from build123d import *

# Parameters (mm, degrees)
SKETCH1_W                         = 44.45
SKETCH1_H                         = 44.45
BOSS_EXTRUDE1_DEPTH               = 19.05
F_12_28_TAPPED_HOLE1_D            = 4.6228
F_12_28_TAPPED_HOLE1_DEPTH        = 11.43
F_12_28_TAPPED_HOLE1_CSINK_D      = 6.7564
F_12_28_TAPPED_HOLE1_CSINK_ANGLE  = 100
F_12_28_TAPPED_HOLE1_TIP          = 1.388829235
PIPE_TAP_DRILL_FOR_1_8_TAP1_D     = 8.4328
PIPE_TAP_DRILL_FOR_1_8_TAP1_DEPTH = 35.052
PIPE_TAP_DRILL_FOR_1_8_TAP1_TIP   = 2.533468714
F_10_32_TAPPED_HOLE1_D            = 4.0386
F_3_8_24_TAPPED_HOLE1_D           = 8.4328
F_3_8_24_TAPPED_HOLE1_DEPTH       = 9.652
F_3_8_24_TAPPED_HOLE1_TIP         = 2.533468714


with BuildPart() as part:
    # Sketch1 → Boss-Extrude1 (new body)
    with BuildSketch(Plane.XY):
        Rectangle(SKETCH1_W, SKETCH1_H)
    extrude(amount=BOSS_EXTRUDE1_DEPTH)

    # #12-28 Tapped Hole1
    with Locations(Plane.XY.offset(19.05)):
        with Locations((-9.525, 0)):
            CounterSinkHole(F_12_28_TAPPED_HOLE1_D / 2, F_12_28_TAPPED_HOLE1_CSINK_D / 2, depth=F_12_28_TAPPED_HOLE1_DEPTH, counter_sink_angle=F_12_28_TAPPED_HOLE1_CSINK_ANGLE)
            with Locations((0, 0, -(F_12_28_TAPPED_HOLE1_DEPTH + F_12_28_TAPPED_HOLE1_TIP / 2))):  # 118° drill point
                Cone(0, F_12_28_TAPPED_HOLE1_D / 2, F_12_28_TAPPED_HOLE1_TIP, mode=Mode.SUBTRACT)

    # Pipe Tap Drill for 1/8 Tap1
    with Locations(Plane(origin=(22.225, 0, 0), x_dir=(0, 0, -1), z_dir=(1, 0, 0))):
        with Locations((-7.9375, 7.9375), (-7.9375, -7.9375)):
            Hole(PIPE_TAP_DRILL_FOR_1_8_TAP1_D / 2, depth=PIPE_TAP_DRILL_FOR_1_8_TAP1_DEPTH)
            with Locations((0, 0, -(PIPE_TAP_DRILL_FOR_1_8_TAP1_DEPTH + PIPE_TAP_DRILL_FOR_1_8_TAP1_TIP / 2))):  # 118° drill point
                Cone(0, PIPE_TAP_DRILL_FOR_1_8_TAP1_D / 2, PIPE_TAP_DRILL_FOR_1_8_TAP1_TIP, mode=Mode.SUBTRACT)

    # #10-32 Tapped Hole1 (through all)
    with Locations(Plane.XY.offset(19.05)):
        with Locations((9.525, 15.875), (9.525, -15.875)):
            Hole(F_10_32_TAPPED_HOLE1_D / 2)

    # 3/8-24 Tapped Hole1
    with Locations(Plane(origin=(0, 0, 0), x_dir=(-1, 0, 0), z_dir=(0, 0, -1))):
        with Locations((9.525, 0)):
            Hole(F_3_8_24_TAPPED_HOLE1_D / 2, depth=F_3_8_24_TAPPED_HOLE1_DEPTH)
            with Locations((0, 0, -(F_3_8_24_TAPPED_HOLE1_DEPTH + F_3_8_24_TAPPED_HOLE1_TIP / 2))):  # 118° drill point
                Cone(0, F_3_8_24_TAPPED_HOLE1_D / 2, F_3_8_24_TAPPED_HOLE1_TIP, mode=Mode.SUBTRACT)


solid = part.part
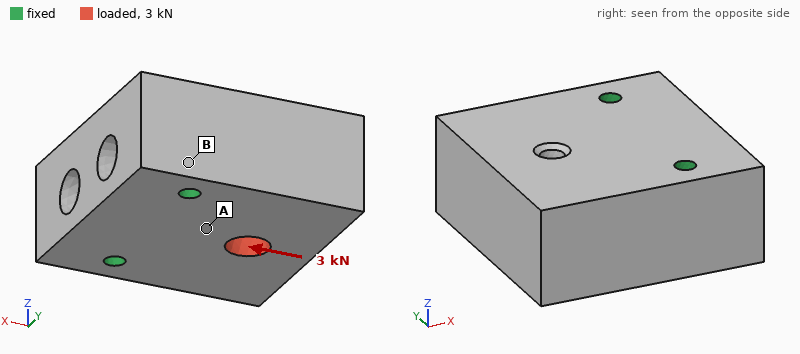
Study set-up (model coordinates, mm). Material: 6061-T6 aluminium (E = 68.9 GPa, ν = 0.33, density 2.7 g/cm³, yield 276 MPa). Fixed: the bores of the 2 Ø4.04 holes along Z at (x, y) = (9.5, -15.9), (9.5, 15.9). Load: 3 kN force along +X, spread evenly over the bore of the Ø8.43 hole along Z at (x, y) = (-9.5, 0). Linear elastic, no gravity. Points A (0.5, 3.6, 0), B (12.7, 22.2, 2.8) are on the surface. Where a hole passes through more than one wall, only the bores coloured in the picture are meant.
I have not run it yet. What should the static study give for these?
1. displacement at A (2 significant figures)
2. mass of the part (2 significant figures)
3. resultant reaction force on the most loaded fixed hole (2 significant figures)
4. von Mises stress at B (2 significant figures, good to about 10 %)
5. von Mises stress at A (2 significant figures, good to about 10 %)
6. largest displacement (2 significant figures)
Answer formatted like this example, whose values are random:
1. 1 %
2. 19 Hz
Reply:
1. 3.8 µm
2. 88 g
3. 1.5 kN
4. 4.7 MPa
5. 11 MPa
6. 8.9 µm
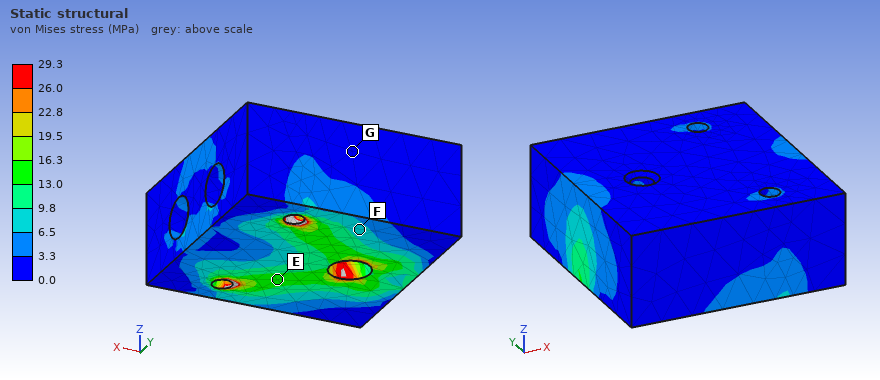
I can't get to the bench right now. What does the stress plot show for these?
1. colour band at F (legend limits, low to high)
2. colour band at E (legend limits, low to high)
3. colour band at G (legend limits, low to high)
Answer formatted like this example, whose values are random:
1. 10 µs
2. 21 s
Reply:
1. 6.5 to 9.8 MPa
2. 13.0 to 16.3 MPa
3. 0.0 to 3.3 MPa
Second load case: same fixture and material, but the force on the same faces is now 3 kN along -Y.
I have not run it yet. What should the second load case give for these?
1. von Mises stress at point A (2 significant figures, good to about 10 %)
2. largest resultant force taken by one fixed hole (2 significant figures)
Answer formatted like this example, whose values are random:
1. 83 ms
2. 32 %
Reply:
1. 17 MPa
2. 2.2 kN
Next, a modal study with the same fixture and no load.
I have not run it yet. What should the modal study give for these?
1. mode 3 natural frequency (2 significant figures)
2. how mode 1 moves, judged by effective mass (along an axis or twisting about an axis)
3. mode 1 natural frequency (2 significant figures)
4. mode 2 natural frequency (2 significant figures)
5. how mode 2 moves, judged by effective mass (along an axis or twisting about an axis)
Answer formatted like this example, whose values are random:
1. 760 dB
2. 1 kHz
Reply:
1. 18 kHz
2. along Z
3. 10 kHz
4. 16 kHz
5. along Y
